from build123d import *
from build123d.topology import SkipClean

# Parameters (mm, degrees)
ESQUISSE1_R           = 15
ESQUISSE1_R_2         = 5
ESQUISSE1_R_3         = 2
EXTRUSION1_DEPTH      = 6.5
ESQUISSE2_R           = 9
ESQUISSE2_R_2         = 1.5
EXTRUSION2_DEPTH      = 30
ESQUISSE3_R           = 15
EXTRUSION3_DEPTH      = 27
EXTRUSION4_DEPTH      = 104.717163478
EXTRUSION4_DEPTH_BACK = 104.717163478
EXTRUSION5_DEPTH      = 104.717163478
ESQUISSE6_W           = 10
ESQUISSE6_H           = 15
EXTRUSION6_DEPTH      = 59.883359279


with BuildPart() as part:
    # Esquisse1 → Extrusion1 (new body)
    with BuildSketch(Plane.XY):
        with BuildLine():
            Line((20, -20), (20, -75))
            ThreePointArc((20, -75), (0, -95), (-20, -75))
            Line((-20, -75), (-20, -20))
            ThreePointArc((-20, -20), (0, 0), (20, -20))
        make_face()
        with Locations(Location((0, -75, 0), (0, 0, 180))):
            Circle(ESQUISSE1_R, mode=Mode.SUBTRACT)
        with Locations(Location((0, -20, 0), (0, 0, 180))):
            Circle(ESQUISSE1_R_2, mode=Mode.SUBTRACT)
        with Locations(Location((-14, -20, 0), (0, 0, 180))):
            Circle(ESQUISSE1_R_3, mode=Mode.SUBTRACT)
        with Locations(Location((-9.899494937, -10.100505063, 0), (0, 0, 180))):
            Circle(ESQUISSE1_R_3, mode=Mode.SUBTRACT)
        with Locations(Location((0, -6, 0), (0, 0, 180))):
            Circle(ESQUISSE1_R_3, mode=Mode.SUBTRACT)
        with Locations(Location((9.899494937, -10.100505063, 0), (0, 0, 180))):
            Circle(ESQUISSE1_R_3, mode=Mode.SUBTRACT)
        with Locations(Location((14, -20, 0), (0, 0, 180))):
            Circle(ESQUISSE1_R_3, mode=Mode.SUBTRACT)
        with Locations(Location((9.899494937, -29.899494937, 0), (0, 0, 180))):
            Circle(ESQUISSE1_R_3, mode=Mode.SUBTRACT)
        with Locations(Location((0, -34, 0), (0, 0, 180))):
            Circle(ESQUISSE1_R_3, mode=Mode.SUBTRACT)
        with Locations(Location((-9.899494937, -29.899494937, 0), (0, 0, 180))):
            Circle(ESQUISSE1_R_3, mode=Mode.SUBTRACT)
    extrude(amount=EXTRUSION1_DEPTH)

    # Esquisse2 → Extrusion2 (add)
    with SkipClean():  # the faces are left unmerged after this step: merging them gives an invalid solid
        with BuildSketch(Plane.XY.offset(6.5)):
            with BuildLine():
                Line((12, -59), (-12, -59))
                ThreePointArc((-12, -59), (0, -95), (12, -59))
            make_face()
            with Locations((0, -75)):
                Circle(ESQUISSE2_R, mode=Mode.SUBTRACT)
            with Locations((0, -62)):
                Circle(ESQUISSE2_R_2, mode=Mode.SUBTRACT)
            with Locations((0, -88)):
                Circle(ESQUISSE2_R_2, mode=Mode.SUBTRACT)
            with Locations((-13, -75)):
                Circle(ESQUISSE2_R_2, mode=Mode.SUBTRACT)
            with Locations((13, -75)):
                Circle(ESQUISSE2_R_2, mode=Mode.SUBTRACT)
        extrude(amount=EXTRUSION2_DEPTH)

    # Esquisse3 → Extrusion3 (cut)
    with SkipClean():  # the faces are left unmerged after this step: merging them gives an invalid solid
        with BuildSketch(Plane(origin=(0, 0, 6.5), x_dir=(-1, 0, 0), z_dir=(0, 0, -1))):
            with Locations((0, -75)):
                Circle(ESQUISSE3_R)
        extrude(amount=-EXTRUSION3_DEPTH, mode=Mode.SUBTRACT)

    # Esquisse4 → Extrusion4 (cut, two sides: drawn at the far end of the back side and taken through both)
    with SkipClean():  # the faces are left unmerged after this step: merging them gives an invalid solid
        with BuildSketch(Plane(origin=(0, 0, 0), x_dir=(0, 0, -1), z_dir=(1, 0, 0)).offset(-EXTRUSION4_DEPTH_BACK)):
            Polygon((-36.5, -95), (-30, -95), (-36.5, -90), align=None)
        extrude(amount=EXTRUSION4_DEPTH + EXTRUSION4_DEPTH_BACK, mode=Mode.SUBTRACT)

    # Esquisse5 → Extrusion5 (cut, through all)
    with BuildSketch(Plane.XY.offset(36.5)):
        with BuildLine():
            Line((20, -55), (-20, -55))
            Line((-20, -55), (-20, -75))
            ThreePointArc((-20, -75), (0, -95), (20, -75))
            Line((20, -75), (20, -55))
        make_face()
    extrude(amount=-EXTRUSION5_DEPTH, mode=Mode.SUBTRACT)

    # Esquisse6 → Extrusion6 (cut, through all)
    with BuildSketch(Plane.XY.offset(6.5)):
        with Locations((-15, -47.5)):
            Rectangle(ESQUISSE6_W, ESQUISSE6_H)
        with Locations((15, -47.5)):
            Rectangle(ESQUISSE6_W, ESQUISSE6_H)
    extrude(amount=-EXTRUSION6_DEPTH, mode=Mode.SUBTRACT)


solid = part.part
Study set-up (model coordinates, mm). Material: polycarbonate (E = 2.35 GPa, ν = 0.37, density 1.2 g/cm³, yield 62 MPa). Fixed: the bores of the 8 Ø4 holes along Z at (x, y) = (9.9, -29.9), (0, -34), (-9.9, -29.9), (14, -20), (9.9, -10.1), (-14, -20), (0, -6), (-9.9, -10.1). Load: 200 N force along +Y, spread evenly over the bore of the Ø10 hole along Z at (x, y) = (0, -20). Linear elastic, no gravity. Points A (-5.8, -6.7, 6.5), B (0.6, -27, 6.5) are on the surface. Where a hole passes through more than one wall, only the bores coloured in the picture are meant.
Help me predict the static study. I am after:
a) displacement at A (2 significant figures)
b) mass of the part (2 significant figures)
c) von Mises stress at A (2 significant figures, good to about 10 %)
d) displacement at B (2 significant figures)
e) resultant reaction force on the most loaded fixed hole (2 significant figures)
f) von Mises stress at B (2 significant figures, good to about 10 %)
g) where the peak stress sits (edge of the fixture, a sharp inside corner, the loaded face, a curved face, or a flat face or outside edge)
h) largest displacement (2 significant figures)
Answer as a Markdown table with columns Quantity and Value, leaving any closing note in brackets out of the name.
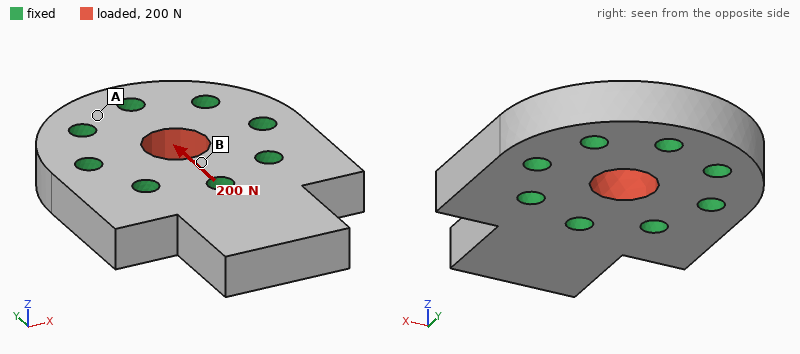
| Quantity | Value |
|---|---|
| displacement at A | 0.64 µm |
| mass of the part | 12 g |
| von Mises stress at A | 0.26 MPa |
| displacement at B | 2.3 µm |
| resultant reaction force on the most loaded fixed hole | 44 N |
| von Mises stress at B | 0.94 MPa |
| where the peak stress sits | the loaded face |
| largest displacement | 3.3 µm |
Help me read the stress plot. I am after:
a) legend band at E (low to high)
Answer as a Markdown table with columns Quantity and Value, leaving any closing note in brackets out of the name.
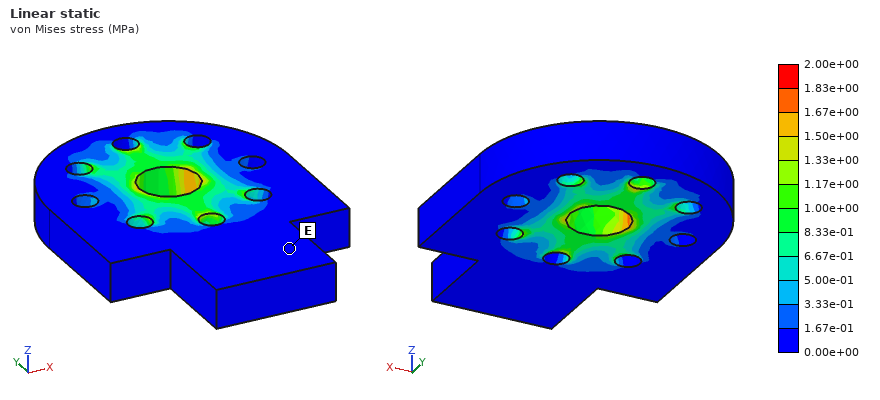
| Quantity | Value |
|---|---|
| legend band at E | 0.00e+00 to 1.67e-01 MPa |
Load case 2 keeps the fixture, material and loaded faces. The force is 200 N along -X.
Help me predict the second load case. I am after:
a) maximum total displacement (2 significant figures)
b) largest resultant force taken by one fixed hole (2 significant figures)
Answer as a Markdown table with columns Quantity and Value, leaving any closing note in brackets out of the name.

| Quantity | Value |
|---|---|
| maximum total displacement | 3.3 µm |
| largest resultant force taken by one fixed hole | 44 N |
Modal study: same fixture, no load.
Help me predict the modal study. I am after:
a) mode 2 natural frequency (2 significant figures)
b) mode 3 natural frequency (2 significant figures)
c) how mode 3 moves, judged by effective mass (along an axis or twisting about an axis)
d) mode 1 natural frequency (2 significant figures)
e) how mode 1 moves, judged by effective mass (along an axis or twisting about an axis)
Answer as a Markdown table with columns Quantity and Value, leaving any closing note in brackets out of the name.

| Quantity | Value |
|---|---|
| mode 2 natural frequency | 6500 Hz |
| mode 3 natural frequency | 7400 Hz |
| how mode 3 moves, judged by effective mass | along X |
| mode 1 natural frequency | 3300 Hz |
| how mode 1 moves, judged by effective mass | along Z |
